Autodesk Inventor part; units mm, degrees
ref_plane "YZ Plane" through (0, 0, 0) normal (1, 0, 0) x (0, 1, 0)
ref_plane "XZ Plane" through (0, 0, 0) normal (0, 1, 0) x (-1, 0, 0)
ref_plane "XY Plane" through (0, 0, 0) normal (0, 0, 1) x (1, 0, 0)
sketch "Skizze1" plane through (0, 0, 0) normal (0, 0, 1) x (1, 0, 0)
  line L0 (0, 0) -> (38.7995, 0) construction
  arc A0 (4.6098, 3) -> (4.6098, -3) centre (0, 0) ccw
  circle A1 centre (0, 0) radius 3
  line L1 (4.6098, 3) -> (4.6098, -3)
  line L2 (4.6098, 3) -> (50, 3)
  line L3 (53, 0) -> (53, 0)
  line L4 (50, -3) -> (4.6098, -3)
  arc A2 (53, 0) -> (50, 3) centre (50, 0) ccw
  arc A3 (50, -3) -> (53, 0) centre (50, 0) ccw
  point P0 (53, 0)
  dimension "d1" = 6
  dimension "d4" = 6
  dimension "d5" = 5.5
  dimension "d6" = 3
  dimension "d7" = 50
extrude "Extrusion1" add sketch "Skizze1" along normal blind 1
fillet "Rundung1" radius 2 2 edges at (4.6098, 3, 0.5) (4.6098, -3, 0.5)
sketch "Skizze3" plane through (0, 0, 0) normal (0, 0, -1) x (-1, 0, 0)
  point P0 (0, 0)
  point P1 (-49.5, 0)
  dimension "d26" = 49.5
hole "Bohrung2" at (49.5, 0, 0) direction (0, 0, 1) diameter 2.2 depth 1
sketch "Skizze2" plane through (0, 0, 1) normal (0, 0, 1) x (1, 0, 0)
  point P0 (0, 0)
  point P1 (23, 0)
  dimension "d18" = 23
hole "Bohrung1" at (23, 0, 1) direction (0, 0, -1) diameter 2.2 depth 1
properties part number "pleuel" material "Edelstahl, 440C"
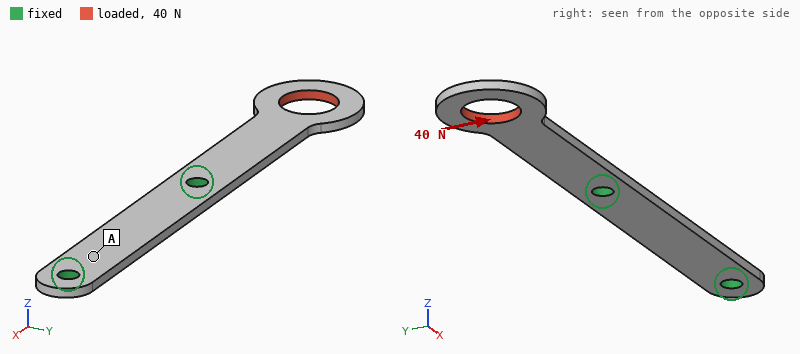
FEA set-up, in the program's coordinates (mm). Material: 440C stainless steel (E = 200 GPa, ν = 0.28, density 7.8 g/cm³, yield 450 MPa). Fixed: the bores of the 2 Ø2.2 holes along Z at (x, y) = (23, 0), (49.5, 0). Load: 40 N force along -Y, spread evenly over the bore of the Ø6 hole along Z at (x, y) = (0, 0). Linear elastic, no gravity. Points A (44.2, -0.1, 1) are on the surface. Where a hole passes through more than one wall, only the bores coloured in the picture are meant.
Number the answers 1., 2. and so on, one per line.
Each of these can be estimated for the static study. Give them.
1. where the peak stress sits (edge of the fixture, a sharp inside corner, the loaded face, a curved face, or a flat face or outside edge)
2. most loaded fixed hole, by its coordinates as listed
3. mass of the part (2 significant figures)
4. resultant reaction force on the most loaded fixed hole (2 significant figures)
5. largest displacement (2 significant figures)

1. edge of the fixture
2. (23, 0)
3. 2.7 g
4. 50 N
5. 77 µm
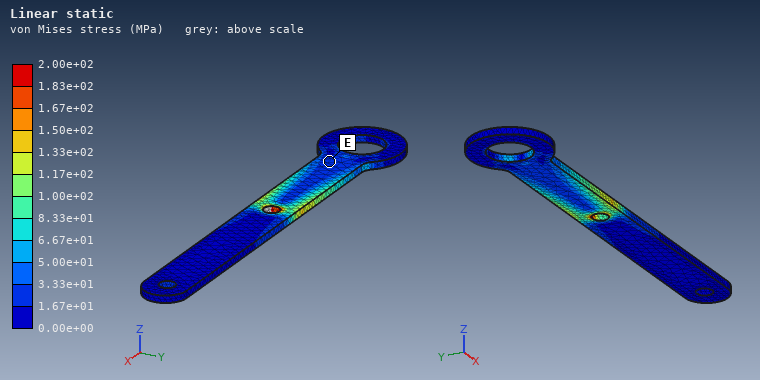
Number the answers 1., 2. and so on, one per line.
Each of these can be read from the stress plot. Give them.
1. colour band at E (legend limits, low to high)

1. 1.67e+01 to 3.33e+01 MPa
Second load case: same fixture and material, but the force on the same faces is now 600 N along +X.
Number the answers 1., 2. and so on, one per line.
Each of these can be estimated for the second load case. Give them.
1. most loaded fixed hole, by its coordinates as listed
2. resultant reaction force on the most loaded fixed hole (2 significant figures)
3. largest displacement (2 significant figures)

1. (23, 0)
2. 590 N
3. 19 µm
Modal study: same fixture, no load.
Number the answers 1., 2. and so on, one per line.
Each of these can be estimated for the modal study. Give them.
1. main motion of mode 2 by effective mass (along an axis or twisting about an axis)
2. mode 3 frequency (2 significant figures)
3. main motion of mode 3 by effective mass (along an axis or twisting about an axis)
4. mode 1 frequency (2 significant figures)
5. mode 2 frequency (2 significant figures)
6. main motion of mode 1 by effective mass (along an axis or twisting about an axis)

1. along Y
2. 5500 Hz
3. twisting about X
4. 1100 Hz
5. 5200 Hz
6. along Z
